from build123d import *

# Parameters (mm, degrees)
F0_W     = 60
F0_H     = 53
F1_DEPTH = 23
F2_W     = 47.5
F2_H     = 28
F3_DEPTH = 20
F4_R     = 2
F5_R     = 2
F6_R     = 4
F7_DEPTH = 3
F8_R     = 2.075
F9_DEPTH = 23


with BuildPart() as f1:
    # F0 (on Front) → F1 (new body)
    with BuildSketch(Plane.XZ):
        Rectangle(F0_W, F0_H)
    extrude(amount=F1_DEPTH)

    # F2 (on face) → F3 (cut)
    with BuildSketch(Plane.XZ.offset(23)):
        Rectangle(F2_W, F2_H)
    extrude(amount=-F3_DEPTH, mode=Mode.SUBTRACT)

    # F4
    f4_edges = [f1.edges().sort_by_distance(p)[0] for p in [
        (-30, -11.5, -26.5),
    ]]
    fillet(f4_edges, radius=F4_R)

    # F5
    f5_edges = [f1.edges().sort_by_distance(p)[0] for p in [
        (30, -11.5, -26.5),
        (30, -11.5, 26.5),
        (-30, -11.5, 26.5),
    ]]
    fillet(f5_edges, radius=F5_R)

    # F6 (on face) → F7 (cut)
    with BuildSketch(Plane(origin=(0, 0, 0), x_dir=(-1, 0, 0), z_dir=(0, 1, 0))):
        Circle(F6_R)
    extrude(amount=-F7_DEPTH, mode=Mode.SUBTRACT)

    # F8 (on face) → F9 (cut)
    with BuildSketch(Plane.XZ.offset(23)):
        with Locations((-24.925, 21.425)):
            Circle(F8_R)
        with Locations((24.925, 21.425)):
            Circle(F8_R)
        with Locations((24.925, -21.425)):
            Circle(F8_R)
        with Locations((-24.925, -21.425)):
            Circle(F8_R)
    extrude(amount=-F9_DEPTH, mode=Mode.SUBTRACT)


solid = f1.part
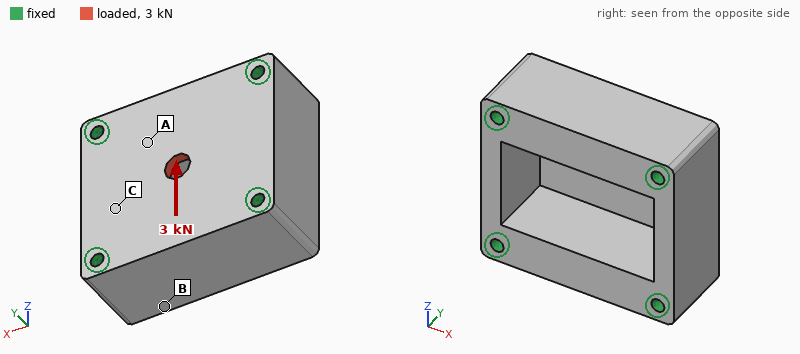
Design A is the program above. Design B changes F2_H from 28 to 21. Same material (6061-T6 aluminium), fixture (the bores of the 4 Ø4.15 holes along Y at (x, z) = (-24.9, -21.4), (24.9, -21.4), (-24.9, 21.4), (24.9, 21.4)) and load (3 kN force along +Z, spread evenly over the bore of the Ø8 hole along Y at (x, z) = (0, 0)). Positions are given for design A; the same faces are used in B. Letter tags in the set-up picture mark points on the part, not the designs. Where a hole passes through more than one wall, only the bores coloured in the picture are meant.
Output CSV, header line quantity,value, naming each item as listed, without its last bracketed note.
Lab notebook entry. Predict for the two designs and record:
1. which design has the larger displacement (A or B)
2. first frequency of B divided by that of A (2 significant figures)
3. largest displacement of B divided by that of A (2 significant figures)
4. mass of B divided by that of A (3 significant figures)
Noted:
quantity,value
which design has the larger displacement,A
first frequency of B divided by that of A,1.1
largest displacement of B divided by that of A,0.92
mass of B divided by that of A,1.15
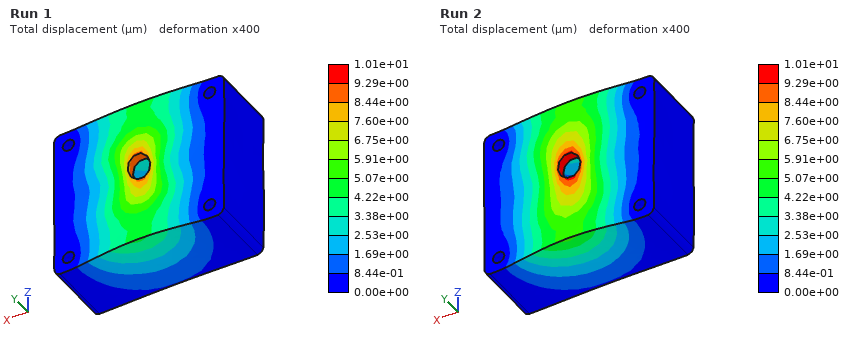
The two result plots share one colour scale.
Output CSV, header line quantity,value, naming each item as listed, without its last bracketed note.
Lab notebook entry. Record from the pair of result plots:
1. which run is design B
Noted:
quantity,value
which run is design B,Run 1
